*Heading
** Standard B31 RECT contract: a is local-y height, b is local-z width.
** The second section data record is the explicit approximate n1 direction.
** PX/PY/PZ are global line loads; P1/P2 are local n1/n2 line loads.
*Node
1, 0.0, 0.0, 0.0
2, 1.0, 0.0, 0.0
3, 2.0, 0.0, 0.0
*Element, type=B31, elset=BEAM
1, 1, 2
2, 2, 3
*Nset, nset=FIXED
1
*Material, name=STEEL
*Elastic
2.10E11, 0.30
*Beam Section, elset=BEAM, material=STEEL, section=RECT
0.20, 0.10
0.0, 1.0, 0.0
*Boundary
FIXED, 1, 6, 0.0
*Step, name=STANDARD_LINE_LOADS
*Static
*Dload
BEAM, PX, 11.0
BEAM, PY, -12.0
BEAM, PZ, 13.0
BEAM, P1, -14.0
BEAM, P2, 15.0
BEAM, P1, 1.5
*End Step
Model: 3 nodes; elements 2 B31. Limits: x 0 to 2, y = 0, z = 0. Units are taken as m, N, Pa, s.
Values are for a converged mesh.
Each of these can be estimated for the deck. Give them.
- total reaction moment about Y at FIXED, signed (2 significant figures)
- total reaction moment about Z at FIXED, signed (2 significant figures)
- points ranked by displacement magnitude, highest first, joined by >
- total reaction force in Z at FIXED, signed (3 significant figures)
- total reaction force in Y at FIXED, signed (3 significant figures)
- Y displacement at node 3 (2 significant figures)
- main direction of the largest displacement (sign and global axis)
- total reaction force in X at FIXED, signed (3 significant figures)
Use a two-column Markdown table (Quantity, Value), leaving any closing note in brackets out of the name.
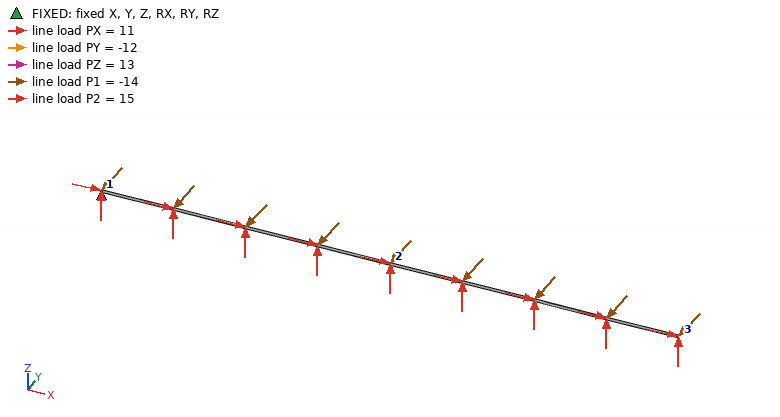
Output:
| Quantity | Value |
|---|---|
| total reaction moment about Y at FIXED, signed | 56 N·m |
| total reaction moment about Z at FIXED, signed | 49 N·m |
| points ranked by displacement magnitude, highest first, joined by > | node 3 > node 2 > node 1 |
| total reaction force in Z at FIXED, signed | -56.0 N |
| total reaction force in Y at FIXED, signed | 49.0 N |
| Y displacement at node 3 | -3.5e-06 m |
| main direction of the largest displacement | +Z |
| total reaction force in X at FIXED, signed | -22.0 N |
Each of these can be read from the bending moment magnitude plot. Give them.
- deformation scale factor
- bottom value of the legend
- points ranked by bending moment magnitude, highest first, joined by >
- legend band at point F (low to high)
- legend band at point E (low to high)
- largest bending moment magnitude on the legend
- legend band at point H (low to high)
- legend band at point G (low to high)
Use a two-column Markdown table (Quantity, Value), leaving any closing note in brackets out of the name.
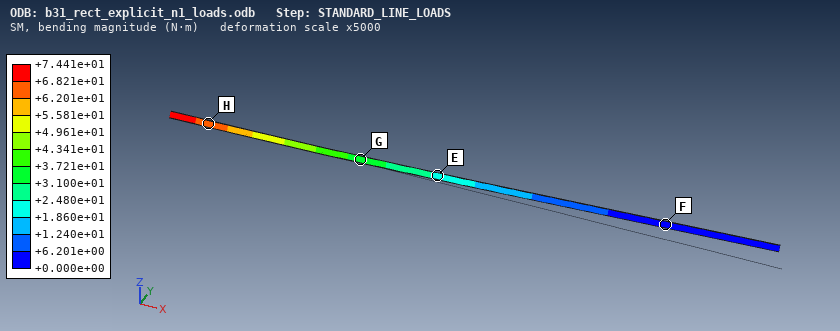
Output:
| Quantity | Value |
|---|---|
| deformation scale factor | 5000 |
| bottom value of the legend | +0.000e+00 N·m |
| points ranked by bending moment magnitude, highest first, joined by > | H > G > E > F |
| legend band at point F | +0.000e+00 to +6.201e+00 N·m |
| legend band at point E | +1.860e+01 to +2.480e+01 N·m |
| largest bending moment magnitude on the legend | +7.441e+01 N·m |
| legend band at point H | +6.201e+01 to +6.821e+01 N·m |
| legend band at point G | +3.100e+01 to +3.721e+01 N·m |
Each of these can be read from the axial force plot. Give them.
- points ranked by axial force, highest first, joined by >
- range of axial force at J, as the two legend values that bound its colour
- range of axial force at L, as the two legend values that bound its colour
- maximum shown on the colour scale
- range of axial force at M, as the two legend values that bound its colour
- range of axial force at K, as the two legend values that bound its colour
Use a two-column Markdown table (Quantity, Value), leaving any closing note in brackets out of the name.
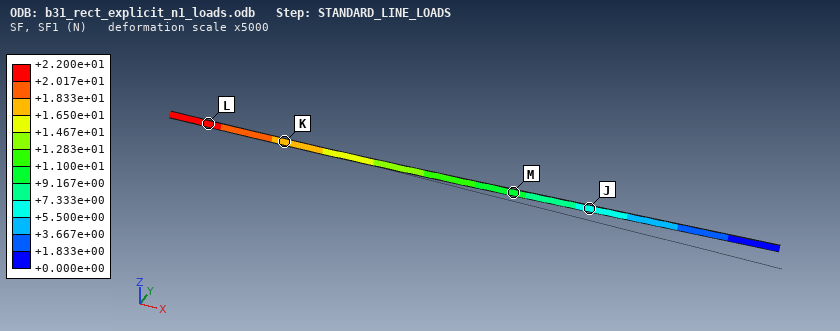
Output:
| Quantity | Value |
|---|---|
| points ranked by axial force, highest first, joined by > | L > K > M > J |
| range of axial force at J, as the two legend values that bound its colour | +5.500e+00 to +7.333e+00 N |
| range of axial force at L, as the two legend values that bound its colour | +2.017e+01 to +2.200e+01 N |
| maximum shown on the colour scale | +2.200e+01 N |
| range of axial force at M, as the two legend values that bound its colour | +9.167e+00 to +1.100e+01 N |
| range of axial force at K, as the two legend values that bound its colour | +1.650e+01 to +1.833e+01 N |
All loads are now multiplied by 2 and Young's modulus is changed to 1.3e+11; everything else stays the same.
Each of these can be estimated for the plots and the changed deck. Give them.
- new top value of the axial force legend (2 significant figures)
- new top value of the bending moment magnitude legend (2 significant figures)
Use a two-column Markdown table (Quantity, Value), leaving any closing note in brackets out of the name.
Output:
| Quantity | Value |
|---|---|
| new top value of the axial force legend | 44 N |
| new top value of the bending moment magnitude legend | 150 N·m |
